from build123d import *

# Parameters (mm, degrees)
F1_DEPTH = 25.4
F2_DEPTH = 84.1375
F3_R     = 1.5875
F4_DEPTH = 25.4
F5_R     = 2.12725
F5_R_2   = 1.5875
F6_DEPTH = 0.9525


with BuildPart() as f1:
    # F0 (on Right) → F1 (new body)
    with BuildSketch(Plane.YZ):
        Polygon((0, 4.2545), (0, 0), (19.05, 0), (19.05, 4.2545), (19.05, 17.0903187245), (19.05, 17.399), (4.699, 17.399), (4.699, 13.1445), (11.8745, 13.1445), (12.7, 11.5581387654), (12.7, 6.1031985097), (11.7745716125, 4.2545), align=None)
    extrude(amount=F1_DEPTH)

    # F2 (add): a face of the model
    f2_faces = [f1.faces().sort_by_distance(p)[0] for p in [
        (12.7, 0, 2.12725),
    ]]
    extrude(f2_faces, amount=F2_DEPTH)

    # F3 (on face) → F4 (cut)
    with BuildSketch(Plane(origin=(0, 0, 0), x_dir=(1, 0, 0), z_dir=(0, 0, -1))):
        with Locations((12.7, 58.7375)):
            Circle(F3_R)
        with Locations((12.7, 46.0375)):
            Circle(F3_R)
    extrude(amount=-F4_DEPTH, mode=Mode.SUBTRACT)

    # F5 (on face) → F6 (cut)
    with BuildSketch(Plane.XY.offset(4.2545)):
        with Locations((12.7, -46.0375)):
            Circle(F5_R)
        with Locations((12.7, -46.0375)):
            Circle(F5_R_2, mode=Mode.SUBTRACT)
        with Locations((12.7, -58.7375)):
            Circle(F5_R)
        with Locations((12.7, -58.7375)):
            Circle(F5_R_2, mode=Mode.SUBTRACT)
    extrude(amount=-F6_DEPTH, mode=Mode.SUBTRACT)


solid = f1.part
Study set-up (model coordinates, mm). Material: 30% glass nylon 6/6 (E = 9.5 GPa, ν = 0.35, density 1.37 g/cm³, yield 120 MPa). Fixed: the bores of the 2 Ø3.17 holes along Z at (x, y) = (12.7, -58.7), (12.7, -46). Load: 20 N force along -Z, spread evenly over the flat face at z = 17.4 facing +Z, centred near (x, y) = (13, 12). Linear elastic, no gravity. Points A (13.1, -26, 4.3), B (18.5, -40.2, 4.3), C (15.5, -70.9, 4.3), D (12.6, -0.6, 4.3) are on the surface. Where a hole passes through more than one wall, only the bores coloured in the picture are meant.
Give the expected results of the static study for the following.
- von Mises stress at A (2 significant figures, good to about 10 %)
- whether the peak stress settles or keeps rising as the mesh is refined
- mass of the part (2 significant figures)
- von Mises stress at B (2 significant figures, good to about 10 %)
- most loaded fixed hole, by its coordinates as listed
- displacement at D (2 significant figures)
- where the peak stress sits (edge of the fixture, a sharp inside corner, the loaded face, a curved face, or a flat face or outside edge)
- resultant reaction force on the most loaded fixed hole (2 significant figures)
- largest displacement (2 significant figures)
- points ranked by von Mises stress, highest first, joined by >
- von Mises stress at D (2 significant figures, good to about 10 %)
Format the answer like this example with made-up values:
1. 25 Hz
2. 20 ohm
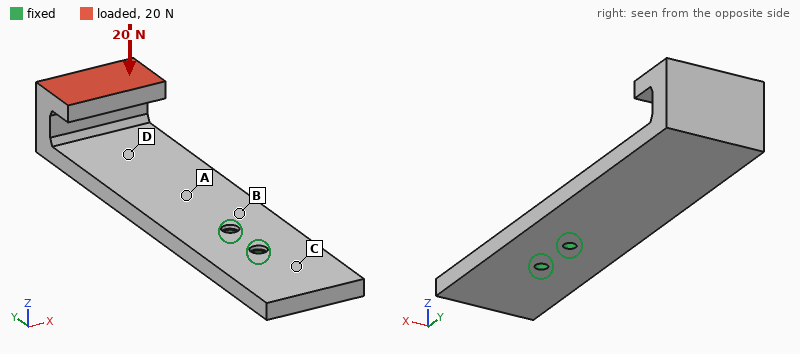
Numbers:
1. 9.3 MPa
2. keeps rising
3. 19 g
4. 13 MPa
5. (12.7, -46)
6. 0.63 mm
7. edge of the fixture
8. 74 N
9. 1.1 mm
10. B > A > D > C
11. 3.3 MPa
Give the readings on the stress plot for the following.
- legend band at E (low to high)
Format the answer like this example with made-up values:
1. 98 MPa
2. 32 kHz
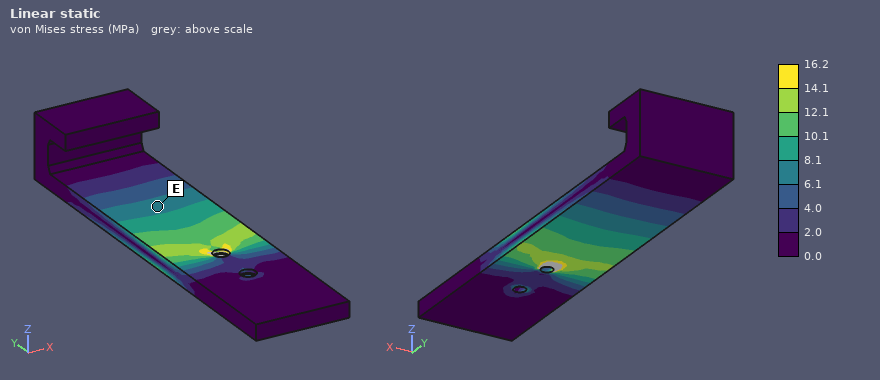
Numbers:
1. 6.1 to 8.1 MPa
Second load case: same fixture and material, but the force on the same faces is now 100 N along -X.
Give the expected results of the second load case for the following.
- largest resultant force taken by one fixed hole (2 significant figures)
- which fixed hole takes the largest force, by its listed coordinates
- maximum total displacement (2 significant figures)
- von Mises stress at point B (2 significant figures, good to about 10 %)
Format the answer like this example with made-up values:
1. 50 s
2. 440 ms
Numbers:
1. 460 N
2. (12.7, -46)
3. 1.1 mm
4. 17 MPa
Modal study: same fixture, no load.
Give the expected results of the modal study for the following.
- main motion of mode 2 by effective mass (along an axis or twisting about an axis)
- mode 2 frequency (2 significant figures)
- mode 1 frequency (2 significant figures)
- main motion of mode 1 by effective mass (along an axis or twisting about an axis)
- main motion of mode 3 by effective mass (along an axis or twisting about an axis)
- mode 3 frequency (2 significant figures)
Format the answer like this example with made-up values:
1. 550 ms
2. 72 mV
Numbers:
1. along X
2. 840 Hz
3. 260 Hz
4. along Z
5. along X
6. 1400 Hz
